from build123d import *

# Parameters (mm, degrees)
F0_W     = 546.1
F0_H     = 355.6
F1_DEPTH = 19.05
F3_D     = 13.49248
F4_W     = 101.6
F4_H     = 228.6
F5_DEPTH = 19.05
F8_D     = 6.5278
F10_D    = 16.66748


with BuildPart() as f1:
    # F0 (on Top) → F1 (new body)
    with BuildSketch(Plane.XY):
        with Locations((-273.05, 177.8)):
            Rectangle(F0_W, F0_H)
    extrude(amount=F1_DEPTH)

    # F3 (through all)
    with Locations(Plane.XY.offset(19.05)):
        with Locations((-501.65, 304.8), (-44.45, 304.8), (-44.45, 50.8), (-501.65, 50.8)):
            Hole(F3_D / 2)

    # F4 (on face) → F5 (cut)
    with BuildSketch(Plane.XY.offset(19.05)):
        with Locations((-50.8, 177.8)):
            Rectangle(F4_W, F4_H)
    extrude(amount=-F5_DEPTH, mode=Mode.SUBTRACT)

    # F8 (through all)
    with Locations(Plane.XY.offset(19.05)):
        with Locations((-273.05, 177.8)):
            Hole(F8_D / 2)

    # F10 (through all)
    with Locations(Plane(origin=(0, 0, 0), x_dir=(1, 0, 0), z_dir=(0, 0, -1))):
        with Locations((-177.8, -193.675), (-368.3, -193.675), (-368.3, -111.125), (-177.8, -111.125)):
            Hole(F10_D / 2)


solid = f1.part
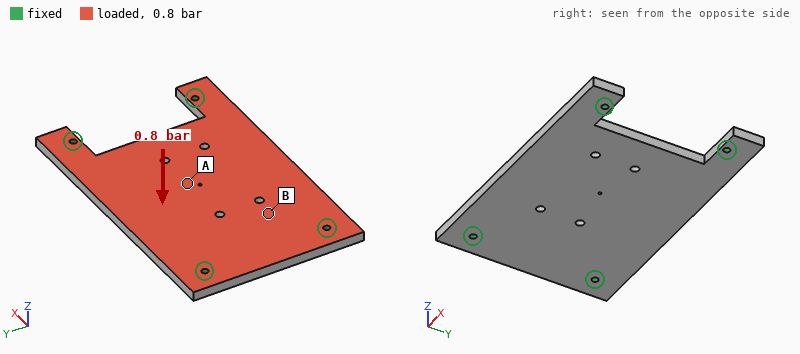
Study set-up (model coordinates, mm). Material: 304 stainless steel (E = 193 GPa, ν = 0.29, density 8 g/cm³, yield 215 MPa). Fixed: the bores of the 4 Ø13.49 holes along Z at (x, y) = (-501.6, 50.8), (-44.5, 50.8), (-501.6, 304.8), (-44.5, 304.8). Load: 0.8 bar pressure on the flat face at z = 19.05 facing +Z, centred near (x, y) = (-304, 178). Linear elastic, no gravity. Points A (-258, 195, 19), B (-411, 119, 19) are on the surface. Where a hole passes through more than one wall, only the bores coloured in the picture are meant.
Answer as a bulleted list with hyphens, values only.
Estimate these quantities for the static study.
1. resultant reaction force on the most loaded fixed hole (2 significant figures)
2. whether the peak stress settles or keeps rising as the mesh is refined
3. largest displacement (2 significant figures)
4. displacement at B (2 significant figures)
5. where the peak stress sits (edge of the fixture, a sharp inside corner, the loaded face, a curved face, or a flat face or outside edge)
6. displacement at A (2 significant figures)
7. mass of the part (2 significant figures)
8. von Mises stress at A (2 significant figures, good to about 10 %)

- 4.0 kN
- keeps rising
- 0.14 mm
- 0.069 mm
- edge of the fixture
- 0.14 mm
- 26 kg
- 12 MPa
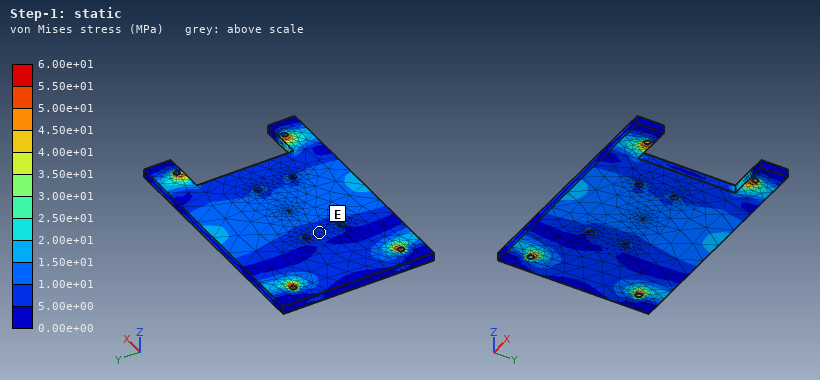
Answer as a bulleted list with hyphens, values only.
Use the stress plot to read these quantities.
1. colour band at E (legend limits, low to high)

- 5.00e+00 to 1.00e+01 MPa
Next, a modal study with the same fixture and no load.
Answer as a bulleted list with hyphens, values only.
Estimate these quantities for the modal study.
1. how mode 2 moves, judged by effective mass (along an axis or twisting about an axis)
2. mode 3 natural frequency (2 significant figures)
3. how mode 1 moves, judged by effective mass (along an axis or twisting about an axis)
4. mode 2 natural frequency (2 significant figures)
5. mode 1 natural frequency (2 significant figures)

- twisting about X
- 870 Hz
- along Z
- 540 Hz
- 350 Hz
